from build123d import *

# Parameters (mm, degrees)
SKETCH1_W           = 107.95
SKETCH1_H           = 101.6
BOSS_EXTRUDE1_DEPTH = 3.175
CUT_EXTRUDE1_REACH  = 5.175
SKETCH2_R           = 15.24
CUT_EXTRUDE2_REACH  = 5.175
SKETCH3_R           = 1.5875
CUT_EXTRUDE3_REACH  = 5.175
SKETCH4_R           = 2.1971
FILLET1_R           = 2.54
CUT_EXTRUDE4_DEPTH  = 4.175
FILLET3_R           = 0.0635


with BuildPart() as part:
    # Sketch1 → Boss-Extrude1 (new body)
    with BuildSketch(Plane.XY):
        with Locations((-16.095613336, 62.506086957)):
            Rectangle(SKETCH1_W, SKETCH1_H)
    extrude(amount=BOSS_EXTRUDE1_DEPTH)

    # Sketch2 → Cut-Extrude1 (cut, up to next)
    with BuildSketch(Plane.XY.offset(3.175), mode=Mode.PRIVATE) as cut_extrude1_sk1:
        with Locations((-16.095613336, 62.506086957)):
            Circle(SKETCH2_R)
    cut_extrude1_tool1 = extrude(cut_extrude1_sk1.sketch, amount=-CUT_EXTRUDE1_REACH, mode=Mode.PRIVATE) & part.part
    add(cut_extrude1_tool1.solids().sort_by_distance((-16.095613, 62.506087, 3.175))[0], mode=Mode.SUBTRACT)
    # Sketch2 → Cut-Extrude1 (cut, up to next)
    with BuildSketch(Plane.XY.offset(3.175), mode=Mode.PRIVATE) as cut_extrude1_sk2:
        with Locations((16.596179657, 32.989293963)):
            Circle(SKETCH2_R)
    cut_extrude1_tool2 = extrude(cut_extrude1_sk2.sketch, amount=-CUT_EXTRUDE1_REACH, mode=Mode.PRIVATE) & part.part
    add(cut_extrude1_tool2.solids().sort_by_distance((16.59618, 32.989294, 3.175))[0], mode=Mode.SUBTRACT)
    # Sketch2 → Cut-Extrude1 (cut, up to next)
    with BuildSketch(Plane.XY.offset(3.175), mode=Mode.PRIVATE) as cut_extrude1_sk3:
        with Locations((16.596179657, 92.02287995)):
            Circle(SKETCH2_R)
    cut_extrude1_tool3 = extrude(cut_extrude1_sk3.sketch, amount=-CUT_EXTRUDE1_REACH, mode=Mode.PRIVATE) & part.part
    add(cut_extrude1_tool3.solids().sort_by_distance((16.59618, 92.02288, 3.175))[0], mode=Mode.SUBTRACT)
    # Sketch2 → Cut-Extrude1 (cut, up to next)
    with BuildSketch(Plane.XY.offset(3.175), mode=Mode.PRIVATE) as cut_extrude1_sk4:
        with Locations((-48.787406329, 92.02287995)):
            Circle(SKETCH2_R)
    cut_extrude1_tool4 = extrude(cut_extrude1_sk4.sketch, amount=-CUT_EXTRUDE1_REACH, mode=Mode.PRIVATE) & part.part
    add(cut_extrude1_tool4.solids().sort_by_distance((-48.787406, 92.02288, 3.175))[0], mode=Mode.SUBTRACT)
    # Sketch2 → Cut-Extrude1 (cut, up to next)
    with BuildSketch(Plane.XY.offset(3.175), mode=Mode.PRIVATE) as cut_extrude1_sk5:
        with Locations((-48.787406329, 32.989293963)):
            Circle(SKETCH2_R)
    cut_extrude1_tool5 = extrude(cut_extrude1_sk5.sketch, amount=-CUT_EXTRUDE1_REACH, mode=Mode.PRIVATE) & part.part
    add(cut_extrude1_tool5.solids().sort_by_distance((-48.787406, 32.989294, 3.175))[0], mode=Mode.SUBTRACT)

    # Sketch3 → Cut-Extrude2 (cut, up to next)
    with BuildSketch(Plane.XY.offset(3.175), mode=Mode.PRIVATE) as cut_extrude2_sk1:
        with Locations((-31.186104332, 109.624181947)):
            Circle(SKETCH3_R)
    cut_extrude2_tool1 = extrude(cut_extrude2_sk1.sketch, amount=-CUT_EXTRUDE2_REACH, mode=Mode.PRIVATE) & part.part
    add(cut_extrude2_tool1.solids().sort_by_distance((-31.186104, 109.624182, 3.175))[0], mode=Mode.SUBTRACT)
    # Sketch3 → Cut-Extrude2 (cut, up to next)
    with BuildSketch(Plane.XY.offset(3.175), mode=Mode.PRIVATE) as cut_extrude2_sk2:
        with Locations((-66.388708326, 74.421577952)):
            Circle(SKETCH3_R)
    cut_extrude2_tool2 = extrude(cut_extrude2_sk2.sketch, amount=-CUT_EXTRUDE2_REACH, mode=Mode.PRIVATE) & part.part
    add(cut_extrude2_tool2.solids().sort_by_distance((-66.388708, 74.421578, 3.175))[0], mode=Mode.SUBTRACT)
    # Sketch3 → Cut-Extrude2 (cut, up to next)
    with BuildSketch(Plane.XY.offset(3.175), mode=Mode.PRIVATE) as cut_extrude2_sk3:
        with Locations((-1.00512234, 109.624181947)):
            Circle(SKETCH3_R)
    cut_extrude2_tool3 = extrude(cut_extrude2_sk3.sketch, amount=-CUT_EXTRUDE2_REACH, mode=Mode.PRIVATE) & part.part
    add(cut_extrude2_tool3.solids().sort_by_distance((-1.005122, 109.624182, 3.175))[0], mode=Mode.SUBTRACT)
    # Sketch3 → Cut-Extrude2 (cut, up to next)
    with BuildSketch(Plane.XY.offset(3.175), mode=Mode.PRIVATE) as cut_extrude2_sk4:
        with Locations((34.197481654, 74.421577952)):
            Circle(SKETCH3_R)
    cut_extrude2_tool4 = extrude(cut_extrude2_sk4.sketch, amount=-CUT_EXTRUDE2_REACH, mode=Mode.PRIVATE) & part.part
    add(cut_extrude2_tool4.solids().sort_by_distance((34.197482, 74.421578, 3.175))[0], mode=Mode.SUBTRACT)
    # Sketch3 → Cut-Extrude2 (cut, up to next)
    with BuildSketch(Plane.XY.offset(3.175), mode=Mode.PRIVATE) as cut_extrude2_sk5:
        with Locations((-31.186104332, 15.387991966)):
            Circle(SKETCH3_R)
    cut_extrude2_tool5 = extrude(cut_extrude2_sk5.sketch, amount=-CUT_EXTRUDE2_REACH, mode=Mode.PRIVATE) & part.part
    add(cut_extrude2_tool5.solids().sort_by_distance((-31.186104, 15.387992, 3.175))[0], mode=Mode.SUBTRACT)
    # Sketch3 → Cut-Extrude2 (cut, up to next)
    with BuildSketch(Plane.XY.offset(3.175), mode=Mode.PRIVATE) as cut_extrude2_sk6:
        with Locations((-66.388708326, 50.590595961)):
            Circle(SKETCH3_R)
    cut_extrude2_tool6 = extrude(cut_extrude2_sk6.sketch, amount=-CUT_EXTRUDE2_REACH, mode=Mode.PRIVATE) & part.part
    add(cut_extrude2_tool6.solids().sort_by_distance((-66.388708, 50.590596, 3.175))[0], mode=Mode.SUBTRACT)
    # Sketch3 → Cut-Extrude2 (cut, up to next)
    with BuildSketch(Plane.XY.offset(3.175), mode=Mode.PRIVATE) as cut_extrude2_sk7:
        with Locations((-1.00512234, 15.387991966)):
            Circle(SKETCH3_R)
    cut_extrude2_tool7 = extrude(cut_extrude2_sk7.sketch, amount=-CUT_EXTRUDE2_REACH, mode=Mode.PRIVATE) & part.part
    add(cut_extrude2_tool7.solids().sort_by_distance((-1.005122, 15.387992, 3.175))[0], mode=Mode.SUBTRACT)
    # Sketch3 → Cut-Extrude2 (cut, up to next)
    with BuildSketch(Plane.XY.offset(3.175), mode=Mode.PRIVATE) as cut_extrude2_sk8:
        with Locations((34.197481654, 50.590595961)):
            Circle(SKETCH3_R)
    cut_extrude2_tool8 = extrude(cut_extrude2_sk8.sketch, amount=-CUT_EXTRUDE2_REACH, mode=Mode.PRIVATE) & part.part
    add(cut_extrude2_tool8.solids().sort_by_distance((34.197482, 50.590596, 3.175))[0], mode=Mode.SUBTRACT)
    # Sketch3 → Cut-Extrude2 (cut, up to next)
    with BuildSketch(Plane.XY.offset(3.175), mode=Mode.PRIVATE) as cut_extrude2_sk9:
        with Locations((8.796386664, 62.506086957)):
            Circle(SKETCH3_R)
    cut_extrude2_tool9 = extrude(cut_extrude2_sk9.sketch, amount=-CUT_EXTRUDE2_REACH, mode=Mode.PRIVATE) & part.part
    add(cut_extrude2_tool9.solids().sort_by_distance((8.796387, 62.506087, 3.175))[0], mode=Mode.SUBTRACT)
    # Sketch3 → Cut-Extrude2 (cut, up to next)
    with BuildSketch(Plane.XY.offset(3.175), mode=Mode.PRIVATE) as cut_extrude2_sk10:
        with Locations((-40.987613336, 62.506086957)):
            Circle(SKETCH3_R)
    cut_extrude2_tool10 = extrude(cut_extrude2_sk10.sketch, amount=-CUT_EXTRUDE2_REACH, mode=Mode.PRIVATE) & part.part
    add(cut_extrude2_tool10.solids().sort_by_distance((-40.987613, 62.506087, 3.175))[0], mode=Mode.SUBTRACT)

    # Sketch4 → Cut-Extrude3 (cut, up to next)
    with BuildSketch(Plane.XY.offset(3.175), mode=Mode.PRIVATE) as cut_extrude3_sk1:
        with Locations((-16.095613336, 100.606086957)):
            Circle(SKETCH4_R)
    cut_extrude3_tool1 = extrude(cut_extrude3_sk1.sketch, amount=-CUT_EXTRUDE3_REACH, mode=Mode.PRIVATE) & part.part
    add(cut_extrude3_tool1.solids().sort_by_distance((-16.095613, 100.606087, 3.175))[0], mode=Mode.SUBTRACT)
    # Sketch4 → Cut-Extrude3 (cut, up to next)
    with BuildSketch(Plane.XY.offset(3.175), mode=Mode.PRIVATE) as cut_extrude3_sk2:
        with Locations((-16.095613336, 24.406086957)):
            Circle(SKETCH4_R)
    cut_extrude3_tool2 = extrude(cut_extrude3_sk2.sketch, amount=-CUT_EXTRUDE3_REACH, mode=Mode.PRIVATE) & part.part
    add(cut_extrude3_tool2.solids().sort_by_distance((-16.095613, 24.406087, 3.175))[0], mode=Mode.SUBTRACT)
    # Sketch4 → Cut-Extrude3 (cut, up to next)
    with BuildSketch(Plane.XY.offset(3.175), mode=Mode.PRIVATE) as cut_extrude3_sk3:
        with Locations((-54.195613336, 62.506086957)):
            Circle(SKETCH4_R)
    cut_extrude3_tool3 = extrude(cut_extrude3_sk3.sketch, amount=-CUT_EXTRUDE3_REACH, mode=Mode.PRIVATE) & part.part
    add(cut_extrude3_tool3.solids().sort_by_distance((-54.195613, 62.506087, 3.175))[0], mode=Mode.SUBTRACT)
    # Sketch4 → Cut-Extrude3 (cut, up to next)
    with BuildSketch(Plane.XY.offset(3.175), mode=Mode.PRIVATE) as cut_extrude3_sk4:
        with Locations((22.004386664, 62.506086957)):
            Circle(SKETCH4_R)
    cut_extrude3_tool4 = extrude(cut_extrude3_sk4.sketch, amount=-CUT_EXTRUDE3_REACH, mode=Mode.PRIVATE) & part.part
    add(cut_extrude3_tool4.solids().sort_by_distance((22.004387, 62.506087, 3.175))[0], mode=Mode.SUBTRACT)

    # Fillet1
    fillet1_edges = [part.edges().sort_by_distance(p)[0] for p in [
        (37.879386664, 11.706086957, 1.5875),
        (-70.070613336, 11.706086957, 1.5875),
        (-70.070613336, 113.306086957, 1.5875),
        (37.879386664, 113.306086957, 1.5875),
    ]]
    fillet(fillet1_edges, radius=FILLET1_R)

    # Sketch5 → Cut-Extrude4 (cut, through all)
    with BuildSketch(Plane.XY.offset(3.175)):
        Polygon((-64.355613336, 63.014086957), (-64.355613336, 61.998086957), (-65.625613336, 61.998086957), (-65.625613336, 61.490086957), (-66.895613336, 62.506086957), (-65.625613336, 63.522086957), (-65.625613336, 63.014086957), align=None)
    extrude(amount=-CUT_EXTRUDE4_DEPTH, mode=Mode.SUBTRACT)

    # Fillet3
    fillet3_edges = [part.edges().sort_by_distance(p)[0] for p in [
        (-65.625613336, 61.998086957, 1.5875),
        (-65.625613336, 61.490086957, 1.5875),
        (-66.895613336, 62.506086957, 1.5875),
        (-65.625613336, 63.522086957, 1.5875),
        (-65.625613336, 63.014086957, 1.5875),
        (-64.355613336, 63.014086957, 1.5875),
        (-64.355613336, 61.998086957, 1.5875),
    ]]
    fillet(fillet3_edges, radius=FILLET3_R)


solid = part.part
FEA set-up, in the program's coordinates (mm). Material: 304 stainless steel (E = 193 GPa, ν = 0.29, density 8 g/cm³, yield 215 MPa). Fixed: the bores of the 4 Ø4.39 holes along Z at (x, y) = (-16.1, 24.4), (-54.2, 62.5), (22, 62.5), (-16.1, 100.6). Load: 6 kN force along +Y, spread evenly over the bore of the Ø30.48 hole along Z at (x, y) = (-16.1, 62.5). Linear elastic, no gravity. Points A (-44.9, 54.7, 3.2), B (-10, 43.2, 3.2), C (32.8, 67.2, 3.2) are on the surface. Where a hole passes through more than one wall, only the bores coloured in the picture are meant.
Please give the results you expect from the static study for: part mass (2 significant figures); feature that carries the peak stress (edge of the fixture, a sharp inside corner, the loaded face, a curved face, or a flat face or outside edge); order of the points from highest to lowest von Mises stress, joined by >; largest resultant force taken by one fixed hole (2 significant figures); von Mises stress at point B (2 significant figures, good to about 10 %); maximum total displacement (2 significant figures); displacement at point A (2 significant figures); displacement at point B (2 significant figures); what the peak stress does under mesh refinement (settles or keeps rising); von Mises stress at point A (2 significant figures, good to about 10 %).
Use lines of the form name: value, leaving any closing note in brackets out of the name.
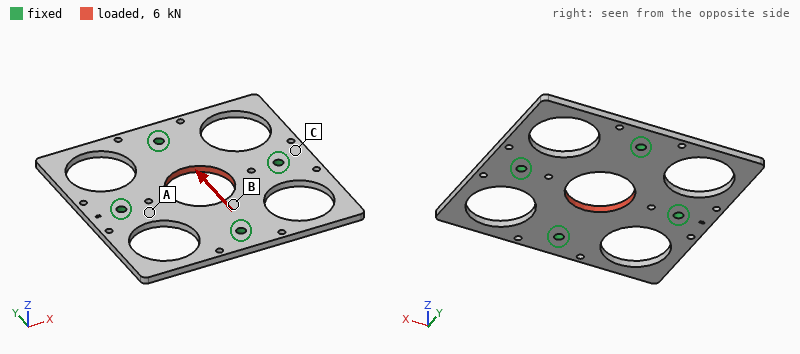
part mass: 180 g
feature that carries the peak stress: edge of the fixture
order of the points from highest to lowest von Mises stress, joined by >: B > A > C
largest resultant force taken by one fixed hole: 2.3 kN
von Mises stress at point B: 31 MPa
maximum total displacement: 5.8 µm
displacement at point A: 2.5 µm
displacement at point B: 3.4 µm
what the peak stress does under mesh refinement: keeps rising
von Mises stress at point A: 15 MPa
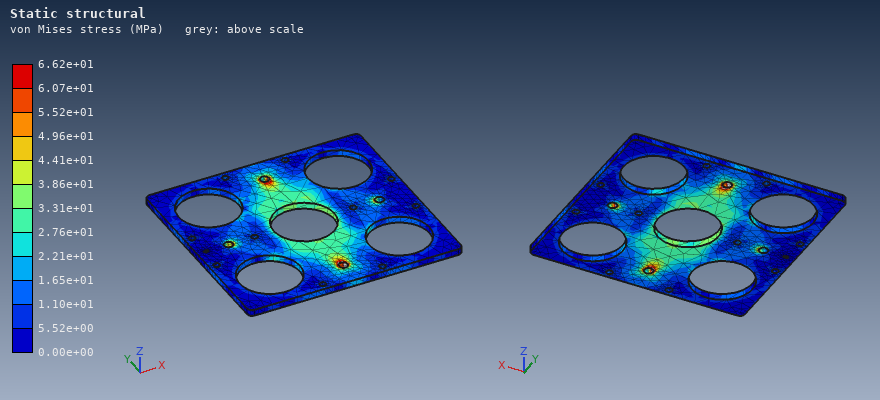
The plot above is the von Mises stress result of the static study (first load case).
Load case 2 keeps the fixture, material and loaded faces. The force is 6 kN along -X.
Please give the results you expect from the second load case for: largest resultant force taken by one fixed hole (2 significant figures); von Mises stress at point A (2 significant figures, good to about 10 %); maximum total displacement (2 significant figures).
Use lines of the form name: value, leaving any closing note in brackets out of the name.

largest resultant force taken by one fixed hole: 2.2 kN
von Mises stress at point A: 24 MPa
maximum total displacement: 5.8 µm
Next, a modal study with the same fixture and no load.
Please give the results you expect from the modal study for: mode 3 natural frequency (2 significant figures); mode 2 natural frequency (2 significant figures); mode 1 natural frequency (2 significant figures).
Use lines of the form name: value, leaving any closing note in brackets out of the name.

mode 3 natural frequency: 1700 Hz
mode 2 natural frequency: 1700 Hz
mode 1 natural frequency: 1600 Hz
